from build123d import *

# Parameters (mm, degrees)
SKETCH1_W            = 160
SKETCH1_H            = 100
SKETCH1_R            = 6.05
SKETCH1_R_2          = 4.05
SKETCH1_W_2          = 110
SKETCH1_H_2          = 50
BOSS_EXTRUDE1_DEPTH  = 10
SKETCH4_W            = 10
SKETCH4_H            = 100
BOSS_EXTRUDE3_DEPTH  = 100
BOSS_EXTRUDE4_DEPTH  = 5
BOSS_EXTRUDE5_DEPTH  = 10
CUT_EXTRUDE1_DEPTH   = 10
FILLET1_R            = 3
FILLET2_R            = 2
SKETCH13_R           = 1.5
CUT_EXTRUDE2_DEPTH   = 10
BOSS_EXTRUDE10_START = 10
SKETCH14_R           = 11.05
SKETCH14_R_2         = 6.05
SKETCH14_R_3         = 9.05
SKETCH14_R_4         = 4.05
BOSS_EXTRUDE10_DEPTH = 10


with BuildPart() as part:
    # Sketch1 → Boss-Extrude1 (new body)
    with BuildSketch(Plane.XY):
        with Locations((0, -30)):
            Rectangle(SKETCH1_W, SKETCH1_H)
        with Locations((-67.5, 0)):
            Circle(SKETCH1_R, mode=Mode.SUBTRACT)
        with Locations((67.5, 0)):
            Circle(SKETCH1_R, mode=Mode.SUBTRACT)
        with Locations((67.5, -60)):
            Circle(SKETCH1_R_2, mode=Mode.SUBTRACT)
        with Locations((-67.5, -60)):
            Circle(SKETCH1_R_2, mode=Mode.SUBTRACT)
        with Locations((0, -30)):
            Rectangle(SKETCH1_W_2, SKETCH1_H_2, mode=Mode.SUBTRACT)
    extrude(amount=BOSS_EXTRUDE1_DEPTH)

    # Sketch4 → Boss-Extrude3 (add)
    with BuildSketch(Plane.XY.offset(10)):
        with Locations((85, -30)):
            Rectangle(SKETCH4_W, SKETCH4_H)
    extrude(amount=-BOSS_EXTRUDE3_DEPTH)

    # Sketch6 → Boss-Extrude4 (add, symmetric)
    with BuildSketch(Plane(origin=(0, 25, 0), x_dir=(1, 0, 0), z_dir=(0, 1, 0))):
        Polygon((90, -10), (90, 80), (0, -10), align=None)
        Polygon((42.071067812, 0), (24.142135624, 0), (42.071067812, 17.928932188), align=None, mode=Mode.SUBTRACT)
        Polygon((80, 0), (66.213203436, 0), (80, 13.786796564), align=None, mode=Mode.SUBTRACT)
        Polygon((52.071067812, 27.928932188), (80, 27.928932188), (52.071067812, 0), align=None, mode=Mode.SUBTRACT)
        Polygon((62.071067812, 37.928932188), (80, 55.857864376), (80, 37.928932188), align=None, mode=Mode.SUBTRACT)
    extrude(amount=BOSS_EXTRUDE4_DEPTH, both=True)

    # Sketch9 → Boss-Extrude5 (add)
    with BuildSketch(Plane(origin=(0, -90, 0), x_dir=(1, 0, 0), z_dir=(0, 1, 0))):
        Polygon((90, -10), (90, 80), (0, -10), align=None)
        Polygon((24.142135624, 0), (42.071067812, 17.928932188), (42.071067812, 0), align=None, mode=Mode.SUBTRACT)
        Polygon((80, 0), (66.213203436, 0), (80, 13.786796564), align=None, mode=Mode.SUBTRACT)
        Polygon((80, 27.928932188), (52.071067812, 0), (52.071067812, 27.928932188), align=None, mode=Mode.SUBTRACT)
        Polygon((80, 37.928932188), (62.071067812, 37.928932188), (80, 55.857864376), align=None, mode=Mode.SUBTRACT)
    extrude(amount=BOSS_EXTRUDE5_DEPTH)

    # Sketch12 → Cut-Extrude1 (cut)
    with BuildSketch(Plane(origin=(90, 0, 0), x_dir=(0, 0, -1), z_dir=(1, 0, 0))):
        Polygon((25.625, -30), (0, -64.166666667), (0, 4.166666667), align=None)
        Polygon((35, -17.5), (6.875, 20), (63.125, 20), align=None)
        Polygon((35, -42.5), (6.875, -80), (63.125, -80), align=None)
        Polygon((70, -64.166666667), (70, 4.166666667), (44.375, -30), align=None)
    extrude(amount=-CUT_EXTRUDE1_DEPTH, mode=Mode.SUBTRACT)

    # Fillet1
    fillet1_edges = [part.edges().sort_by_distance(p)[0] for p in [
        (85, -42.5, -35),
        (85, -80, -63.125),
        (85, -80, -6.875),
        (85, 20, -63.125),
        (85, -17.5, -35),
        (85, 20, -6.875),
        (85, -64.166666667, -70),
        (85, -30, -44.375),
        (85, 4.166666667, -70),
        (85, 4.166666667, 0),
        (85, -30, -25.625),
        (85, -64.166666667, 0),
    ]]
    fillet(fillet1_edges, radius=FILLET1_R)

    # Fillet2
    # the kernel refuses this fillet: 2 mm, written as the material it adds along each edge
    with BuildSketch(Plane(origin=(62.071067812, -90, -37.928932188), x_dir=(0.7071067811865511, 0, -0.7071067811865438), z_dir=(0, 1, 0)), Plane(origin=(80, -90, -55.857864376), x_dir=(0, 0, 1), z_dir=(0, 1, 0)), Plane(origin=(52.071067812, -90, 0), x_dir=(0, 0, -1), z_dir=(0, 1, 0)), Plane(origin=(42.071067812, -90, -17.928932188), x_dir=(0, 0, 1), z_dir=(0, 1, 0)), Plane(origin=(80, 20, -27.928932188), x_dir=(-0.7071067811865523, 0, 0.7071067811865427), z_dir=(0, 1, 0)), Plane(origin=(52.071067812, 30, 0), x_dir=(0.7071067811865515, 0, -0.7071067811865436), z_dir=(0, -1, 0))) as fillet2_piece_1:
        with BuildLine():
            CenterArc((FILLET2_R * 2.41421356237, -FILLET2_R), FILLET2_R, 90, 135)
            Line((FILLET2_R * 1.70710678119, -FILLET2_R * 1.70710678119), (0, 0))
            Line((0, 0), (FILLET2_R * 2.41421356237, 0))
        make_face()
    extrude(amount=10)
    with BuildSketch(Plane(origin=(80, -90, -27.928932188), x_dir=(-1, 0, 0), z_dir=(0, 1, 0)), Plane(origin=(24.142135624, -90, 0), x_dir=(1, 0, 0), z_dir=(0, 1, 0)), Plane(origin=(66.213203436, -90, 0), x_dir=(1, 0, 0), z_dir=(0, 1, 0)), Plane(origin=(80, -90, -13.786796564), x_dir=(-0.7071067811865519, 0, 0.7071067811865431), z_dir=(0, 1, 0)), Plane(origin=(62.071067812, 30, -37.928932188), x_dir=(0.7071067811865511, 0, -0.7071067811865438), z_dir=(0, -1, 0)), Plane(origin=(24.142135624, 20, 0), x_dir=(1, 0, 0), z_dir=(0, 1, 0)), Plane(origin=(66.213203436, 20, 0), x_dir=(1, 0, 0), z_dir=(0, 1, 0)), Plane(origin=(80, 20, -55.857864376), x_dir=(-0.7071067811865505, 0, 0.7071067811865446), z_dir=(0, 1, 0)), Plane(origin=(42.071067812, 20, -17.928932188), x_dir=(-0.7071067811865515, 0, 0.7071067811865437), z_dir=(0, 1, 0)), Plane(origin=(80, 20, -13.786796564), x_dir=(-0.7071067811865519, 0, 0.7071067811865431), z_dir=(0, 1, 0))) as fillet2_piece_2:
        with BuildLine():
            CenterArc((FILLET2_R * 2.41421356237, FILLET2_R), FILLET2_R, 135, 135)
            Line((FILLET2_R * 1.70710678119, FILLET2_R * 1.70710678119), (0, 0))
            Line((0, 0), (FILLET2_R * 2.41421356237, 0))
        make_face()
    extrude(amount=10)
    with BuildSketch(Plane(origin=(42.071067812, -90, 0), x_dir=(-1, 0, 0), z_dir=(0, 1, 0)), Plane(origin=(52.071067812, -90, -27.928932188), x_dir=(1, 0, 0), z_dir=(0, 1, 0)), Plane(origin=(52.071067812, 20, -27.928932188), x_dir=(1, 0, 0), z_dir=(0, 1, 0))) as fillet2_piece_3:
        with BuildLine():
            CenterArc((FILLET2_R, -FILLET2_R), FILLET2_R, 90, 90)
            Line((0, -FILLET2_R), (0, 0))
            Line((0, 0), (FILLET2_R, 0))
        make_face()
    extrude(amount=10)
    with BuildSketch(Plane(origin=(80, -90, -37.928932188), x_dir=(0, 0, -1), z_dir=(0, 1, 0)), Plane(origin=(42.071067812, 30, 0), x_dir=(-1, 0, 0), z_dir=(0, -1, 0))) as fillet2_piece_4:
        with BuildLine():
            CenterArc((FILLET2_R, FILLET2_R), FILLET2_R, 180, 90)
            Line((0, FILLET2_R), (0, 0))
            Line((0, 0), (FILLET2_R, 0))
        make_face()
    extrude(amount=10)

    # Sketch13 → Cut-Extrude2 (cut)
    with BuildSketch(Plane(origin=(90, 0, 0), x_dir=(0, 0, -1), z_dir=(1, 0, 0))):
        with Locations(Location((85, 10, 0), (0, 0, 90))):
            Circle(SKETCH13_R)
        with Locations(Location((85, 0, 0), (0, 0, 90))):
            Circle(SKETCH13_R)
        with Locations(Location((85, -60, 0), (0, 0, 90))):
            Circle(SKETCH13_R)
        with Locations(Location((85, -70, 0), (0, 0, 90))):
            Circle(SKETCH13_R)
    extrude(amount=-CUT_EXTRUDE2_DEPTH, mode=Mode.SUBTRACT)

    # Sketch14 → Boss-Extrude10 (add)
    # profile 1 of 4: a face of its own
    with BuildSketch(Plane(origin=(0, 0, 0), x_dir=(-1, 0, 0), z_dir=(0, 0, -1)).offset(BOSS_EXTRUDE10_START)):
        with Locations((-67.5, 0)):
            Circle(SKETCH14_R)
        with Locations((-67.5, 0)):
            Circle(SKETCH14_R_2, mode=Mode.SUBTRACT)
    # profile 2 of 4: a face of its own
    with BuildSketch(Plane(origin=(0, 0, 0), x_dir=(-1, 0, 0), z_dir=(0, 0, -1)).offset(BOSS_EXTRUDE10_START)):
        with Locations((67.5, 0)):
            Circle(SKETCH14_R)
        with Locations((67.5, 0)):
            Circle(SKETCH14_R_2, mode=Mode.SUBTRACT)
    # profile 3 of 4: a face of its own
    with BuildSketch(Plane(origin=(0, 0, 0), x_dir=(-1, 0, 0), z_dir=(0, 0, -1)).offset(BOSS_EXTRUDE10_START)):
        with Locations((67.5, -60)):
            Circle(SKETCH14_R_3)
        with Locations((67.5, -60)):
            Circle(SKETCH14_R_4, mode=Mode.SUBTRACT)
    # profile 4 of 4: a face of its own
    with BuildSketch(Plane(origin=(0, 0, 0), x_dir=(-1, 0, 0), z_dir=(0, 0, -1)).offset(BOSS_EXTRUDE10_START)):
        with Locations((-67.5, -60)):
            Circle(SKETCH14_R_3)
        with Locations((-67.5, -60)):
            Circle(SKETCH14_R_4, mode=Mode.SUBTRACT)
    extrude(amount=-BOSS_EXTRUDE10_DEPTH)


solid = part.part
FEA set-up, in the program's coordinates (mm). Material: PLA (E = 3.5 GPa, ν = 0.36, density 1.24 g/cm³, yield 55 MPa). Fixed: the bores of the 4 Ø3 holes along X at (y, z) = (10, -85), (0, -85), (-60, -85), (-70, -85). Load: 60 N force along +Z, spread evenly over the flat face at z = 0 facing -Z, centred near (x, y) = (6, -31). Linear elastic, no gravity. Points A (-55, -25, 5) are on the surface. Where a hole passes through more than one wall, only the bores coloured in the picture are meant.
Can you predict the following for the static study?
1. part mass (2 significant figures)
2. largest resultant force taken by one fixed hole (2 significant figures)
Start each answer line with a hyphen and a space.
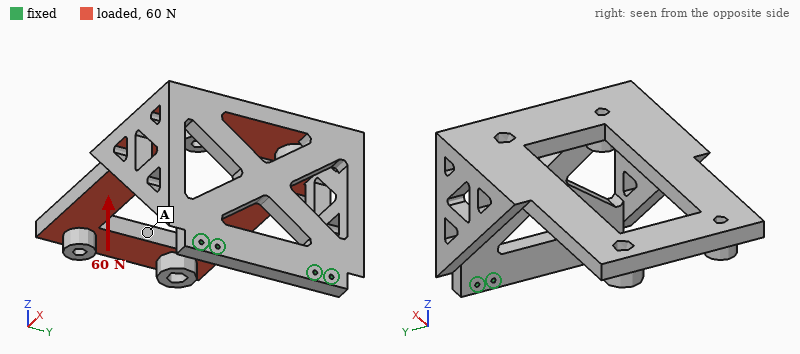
- 300 g
- 46 N
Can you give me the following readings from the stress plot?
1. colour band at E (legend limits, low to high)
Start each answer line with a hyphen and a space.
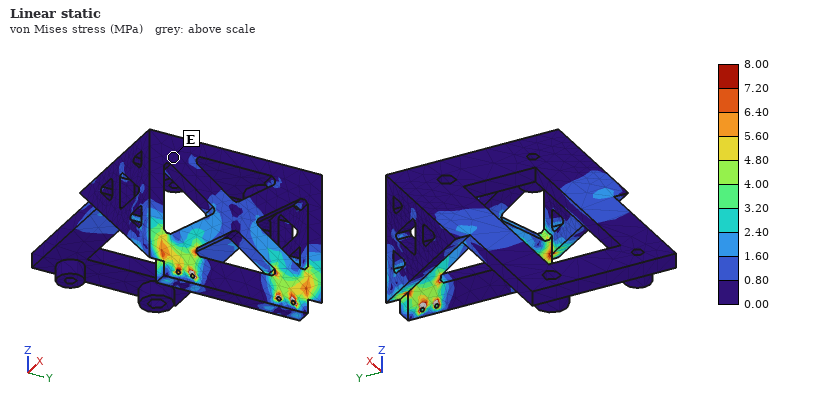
- 0.00 to 0.80 MPa
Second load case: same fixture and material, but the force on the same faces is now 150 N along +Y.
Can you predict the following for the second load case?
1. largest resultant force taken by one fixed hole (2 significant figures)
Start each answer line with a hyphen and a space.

- 230 N
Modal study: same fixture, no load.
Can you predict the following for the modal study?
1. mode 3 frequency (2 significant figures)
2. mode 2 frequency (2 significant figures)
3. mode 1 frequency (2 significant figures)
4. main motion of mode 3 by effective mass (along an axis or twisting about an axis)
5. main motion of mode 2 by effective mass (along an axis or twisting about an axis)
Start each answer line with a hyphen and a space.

- 230 Hz
- 110 Hz
- 63 Hz
- along X
- along Y
